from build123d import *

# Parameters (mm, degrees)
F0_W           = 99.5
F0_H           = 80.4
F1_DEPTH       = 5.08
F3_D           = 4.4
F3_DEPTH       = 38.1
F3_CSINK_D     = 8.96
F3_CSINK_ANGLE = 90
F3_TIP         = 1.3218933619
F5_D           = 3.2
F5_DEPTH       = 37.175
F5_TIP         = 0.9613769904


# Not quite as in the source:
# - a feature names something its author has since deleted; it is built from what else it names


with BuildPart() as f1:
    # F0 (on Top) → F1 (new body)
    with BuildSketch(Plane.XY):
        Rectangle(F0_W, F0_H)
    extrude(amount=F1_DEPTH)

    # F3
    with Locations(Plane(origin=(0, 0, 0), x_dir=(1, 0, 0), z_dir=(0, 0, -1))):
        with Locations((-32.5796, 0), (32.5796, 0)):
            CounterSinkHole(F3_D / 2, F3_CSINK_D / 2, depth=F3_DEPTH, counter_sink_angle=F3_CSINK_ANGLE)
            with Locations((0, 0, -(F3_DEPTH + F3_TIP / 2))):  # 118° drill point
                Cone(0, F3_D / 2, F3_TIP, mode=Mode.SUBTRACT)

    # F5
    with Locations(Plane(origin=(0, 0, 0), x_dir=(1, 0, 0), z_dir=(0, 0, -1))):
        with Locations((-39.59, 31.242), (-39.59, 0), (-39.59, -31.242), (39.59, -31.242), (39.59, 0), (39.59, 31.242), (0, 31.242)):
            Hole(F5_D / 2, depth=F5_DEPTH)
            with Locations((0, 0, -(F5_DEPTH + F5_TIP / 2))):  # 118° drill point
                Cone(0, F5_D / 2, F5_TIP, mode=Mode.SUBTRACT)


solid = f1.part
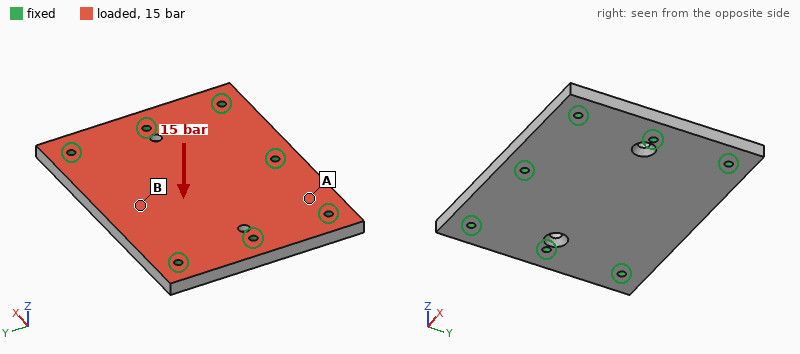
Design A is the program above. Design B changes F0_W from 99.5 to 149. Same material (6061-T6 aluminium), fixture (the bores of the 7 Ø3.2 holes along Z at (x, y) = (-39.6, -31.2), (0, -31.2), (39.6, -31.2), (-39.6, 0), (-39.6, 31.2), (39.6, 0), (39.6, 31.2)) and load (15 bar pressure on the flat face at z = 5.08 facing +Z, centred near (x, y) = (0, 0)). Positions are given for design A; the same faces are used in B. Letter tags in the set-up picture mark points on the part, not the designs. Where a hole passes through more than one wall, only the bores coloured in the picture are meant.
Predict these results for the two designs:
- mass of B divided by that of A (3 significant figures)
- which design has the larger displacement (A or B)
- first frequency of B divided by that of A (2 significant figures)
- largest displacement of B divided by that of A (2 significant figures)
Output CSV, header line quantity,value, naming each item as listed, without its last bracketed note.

quantity,value
mass of B divided by that of A,1.50
which design has the larger displacement,B
first frequency of B divided by that of A,0.73
largest displacement of B divided by that of A,1.5
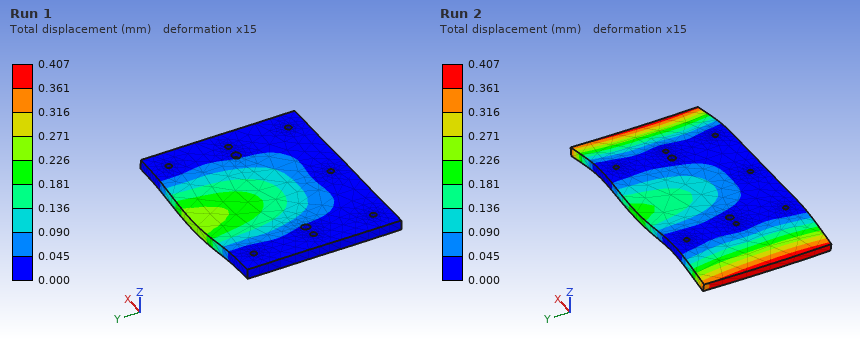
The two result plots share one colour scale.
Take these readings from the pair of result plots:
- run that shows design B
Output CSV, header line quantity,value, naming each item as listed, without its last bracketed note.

quantity,value
run that shows design B,Run 2
